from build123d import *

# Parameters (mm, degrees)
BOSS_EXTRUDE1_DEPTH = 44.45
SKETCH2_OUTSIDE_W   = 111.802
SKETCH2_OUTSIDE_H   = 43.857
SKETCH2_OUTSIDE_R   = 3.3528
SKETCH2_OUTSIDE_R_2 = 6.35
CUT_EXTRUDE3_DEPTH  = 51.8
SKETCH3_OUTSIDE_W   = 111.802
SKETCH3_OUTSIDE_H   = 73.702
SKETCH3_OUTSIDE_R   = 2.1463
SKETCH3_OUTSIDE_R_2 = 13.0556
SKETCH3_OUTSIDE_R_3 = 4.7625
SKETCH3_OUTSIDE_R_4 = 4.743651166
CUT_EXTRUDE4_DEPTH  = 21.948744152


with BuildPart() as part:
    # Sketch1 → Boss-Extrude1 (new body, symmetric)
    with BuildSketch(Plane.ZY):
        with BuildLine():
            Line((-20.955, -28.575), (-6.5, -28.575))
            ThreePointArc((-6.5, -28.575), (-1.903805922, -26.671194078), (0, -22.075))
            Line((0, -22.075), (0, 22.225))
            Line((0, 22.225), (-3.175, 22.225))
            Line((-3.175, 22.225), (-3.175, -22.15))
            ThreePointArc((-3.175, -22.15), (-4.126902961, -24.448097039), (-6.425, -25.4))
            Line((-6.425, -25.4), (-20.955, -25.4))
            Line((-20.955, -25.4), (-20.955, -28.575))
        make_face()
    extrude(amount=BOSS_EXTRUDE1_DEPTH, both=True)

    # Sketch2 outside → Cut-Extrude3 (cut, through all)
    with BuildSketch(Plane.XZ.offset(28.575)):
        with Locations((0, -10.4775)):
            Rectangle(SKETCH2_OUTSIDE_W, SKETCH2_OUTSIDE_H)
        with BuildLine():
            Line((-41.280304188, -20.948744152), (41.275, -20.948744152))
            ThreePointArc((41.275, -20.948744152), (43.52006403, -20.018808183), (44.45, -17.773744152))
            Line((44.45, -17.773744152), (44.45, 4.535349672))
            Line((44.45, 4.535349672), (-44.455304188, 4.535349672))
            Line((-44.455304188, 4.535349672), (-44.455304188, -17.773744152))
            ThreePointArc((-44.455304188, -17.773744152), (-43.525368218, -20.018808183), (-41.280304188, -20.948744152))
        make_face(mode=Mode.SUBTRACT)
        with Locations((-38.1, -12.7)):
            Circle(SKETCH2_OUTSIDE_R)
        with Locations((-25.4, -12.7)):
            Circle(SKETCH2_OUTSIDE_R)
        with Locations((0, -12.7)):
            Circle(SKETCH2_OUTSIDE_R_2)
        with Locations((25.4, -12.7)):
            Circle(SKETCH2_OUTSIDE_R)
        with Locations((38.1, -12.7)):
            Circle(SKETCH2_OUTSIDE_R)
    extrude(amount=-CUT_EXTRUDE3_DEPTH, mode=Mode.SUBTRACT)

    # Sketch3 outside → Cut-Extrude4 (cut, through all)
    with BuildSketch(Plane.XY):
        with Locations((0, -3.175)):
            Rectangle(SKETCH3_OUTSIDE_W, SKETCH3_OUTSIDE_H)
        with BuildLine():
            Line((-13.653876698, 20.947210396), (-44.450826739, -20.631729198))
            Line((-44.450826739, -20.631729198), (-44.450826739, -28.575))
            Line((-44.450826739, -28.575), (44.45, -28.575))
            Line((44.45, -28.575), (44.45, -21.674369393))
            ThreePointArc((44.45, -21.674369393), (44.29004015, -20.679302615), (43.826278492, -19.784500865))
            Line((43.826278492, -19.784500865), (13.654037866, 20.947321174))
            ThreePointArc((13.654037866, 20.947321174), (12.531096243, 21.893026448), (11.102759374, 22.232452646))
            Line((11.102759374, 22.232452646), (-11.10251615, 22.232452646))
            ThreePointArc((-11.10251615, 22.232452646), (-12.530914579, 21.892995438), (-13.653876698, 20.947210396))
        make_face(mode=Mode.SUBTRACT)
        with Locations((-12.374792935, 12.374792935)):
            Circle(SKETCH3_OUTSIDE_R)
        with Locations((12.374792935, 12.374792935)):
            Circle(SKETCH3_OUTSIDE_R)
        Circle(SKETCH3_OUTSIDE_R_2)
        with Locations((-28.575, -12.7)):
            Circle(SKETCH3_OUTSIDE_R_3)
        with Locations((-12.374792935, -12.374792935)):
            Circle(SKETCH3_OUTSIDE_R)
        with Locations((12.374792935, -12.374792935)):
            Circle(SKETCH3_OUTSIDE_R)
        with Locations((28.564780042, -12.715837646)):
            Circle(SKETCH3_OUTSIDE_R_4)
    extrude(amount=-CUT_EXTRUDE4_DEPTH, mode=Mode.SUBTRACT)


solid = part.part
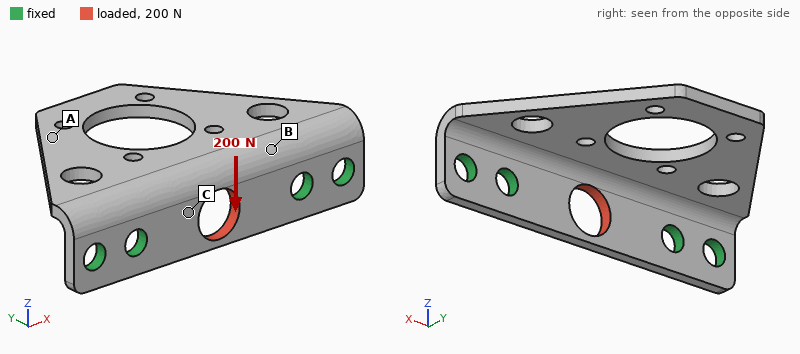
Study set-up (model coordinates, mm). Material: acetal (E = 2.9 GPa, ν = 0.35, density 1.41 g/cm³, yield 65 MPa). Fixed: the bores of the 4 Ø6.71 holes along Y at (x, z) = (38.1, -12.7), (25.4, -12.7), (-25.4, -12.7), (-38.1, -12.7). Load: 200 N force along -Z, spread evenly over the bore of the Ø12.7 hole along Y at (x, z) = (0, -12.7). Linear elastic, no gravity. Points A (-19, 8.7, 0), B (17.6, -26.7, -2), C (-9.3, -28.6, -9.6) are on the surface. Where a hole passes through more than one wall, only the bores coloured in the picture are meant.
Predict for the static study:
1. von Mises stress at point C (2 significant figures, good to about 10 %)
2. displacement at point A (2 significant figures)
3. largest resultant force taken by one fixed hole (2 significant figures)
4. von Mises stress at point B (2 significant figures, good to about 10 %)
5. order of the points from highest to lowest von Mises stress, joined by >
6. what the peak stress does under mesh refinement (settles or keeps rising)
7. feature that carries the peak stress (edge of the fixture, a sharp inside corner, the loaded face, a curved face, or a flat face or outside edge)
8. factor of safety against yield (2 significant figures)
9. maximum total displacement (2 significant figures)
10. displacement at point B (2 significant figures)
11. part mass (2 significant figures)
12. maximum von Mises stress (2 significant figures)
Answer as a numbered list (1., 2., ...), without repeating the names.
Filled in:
1. 4.0 MPa
2. 16 µm
3. 130 N
4. 2.2 MPa
5. C > B > A
6. settles
7. a flat face or outside edge
8. 4.7
9. 84 µm
10. 23 µm
11. 16 g
12. 14 MPa
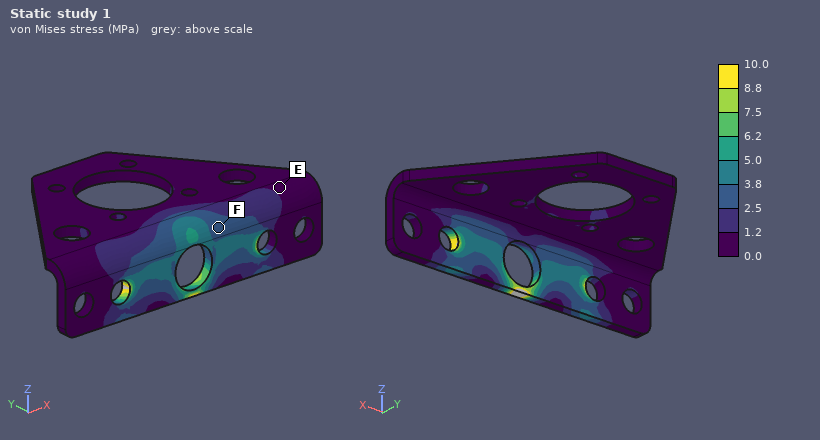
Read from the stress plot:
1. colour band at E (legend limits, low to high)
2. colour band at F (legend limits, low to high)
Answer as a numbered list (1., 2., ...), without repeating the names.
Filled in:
1. 0.0 to 1.2 MPa
2. 2.5 to 3.8 MPa
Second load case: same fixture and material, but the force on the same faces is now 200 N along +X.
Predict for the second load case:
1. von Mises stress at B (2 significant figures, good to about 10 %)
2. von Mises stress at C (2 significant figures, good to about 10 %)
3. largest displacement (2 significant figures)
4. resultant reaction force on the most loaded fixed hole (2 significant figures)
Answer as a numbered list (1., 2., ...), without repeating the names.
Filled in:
1. 0.60 MPa
2. 1.8 MPa
3. 17 µm
4. 86 N
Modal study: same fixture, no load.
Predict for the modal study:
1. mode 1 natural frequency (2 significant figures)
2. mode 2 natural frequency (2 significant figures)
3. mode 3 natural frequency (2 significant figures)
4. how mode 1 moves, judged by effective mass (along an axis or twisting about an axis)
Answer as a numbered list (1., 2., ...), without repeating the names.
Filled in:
1. 330 Hz
2. 830 Hz
3. 1400 Hz
4. along Z
